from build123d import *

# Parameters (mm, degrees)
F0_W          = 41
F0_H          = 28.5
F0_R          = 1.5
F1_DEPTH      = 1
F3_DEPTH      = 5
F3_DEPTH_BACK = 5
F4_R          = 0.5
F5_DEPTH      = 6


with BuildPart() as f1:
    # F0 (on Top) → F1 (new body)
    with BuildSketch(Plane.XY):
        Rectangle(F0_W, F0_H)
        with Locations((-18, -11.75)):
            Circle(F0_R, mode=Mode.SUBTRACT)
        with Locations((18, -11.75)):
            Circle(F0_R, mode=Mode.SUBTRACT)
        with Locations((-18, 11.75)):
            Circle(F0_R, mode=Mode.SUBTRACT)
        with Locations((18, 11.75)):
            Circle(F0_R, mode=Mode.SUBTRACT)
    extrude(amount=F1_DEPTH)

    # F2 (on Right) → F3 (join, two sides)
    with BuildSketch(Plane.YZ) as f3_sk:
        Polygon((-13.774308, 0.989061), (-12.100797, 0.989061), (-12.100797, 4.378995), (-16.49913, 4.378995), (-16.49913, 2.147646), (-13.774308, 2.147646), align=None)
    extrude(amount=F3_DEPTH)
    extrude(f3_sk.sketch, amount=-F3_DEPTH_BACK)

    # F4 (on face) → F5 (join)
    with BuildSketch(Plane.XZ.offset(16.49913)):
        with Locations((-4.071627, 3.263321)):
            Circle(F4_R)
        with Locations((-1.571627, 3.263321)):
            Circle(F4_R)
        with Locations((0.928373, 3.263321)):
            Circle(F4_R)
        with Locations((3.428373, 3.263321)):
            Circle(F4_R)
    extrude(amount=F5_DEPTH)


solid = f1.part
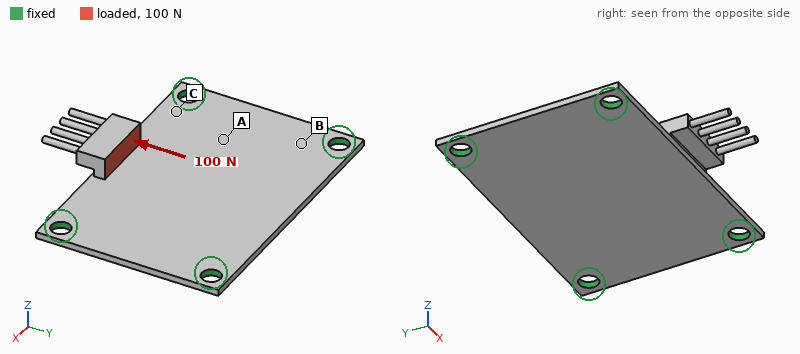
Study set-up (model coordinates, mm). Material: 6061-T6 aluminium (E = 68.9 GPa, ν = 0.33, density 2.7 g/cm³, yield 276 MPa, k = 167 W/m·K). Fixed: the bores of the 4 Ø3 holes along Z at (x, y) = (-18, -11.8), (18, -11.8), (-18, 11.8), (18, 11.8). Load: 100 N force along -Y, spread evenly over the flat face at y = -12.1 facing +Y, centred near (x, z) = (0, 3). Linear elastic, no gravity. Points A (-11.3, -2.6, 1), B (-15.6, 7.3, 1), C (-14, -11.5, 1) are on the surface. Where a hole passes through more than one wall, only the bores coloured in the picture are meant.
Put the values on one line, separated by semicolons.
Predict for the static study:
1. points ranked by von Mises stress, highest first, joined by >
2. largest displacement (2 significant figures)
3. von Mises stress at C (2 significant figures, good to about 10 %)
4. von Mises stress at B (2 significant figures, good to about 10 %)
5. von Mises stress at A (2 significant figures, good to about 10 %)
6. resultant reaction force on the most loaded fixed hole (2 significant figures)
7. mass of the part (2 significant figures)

C > A > B; 0.16 mm; 35 MPa; 5.7 MPa; 13 MPa; 33 N; 3.4 g
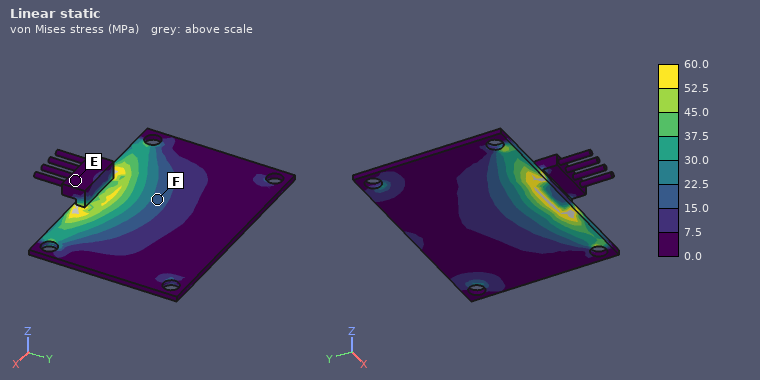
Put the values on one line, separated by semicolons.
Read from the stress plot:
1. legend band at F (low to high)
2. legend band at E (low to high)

15.0 to 22.5 MPa; 0.0 to 7.5 MPa
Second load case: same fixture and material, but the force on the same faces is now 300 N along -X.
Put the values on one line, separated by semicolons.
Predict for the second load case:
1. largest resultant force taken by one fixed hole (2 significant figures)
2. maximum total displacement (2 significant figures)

120 N; 72 µm
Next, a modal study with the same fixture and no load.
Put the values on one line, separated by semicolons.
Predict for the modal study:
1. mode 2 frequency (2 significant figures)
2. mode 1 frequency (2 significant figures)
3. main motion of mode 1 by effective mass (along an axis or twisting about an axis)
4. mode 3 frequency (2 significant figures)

4400 Hz; 3600 Hz; along Z; 7300 Hz
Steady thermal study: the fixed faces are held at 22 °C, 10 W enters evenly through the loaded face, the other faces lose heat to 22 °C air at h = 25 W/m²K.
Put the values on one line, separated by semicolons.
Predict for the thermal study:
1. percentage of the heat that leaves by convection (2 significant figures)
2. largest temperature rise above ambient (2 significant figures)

8.1 %; 44 K
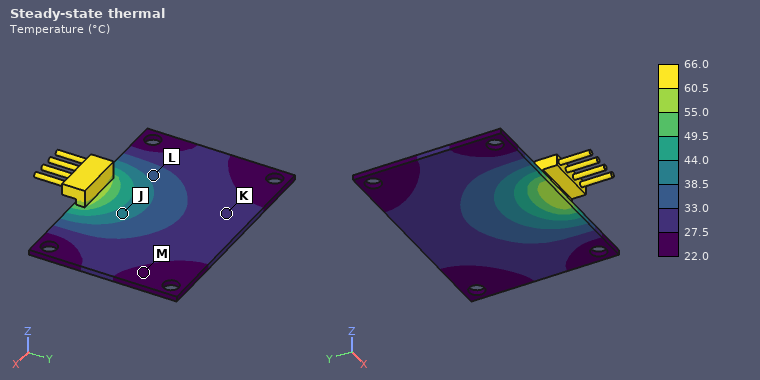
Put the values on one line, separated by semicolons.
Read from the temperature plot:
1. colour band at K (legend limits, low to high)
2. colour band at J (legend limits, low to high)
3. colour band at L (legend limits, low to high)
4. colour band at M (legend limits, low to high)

27.5 to 33.0 °C; 38.5 to 44.0 °C; 33.0 to 38.5 °C; 22.0 to 27.5 °C
